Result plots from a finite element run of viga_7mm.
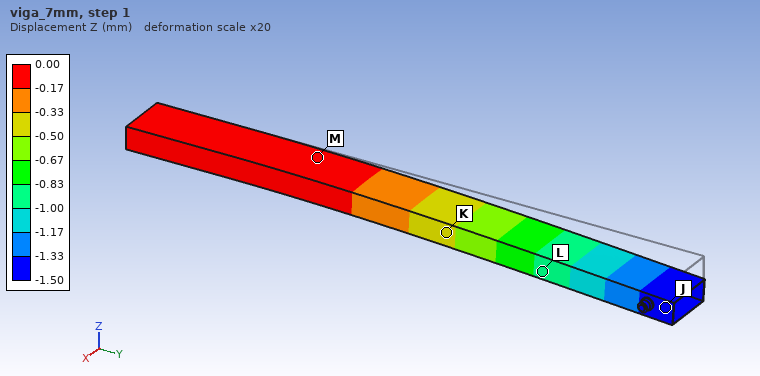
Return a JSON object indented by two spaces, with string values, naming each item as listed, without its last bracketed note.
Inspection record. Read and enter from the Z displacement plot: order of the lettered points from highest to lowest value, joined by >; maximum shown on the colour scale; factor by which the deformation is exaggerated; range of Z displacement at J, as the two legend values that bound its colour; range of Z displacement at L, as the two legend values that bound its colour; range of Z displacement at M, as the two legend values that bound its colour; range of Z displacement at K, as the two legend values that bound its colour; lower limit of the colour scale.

{
  "order of the lettered points from highest to lowest value, joined by >": "M > K > L > J",
  "maximum shown on the colour scale": "0.00 mm",
  "factor by which the deformation is exaggerated": "20",
  "range of Z displacement at J, as the two legend values that bound its colour": "-1.50 to -1.33 mm",
  "range of Z displacement at L, as the two legend values that bound its colour": "-1.00 to -0.83 mm",
  "range of Z displacement at M, as the two legend values that bound its colour": "-0.17 to 0.00 mm",
  "range of Z displacement at K, as the two legend values that bound its colour": "-0.50 to -0.33 mm",
  "lower limit of the colour scale": "-1.50 mm"
}
